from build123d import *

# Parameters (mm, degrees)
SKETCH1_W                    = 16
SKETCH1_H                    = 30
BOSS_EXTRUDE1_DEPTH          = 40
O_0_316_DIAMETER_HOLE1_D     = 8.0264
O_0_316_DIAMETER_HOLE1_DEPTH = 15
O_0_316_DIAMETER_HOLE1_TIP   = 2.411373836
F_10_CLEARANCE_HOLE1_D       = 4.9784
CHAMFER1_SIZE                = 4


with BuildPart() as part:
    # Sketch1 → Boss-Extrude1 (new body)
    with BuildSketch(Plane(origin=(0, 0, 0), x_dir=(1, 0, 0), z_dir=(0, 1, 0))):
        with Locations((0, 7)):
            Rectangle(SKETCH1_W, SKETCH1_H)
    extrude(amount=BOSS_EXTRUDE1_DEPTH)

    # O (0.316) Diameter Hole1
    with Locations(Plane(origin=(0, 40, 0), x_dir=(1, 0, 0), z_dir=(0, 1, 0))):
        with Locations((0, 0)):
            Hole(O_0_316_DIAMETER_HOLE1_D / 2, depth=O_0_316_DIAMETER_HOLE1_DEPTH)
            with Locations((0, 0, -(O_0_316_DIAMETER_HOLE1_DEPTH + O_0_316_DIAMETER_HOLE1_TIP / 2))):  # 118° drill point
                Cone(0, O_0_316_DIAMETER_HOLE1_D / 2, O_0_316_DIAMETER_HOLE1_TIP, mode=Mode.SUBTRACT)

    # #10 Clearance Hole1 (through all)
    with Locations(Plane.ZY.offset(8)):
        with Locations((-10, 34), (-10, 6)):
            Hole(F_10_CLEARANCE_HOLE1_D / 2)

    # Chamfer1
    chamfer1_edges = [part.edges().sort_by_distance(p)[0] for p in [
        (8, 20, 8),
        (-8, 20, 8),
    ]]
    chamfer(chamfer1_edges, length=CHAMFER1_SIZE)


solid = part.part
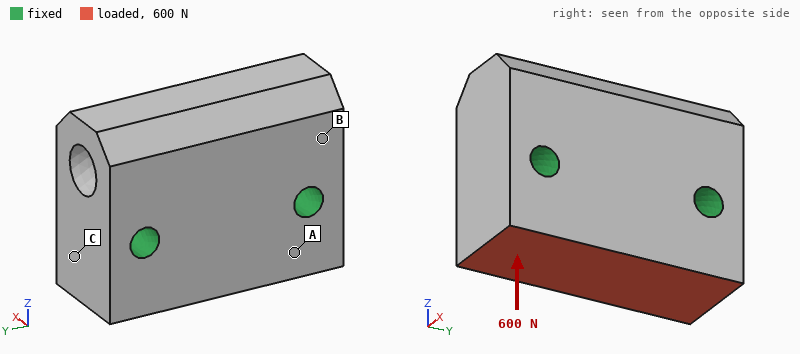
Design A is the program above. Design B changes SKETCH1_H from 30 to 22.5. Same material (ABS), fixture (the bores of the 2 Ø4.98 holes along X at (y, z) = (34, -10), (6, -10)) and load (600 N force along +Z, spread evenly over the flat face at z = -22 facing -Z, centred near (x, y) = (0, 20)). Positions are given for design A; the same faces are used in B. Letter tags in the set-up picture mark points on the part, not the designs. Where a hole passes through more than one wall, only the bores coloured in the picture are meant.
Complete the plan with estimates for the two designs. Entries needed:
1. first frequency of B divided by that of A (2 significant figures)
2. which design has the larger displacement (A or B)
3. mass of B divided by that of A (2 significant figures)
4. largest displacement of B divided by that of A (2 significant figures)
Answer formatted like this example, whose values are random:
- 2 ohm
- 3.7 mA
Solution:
- 1.4
- B
- 0.72
- 1.1
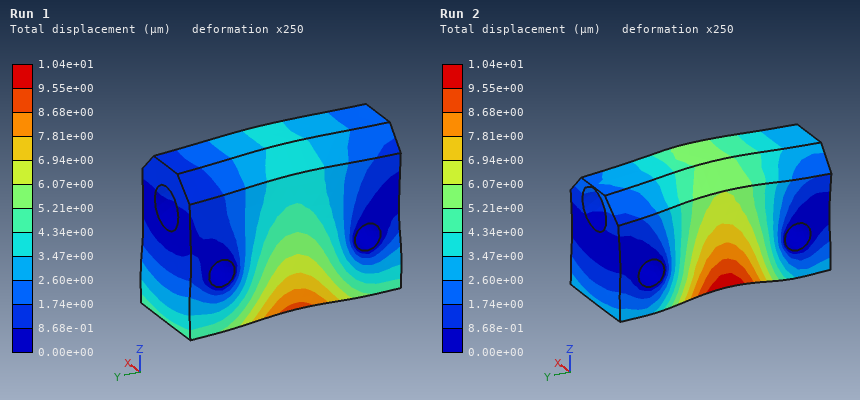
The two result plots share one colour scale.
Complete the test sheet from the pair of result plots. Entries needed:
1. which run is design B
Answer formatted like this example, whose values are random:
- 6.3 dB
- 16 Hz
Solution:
- Run 2
